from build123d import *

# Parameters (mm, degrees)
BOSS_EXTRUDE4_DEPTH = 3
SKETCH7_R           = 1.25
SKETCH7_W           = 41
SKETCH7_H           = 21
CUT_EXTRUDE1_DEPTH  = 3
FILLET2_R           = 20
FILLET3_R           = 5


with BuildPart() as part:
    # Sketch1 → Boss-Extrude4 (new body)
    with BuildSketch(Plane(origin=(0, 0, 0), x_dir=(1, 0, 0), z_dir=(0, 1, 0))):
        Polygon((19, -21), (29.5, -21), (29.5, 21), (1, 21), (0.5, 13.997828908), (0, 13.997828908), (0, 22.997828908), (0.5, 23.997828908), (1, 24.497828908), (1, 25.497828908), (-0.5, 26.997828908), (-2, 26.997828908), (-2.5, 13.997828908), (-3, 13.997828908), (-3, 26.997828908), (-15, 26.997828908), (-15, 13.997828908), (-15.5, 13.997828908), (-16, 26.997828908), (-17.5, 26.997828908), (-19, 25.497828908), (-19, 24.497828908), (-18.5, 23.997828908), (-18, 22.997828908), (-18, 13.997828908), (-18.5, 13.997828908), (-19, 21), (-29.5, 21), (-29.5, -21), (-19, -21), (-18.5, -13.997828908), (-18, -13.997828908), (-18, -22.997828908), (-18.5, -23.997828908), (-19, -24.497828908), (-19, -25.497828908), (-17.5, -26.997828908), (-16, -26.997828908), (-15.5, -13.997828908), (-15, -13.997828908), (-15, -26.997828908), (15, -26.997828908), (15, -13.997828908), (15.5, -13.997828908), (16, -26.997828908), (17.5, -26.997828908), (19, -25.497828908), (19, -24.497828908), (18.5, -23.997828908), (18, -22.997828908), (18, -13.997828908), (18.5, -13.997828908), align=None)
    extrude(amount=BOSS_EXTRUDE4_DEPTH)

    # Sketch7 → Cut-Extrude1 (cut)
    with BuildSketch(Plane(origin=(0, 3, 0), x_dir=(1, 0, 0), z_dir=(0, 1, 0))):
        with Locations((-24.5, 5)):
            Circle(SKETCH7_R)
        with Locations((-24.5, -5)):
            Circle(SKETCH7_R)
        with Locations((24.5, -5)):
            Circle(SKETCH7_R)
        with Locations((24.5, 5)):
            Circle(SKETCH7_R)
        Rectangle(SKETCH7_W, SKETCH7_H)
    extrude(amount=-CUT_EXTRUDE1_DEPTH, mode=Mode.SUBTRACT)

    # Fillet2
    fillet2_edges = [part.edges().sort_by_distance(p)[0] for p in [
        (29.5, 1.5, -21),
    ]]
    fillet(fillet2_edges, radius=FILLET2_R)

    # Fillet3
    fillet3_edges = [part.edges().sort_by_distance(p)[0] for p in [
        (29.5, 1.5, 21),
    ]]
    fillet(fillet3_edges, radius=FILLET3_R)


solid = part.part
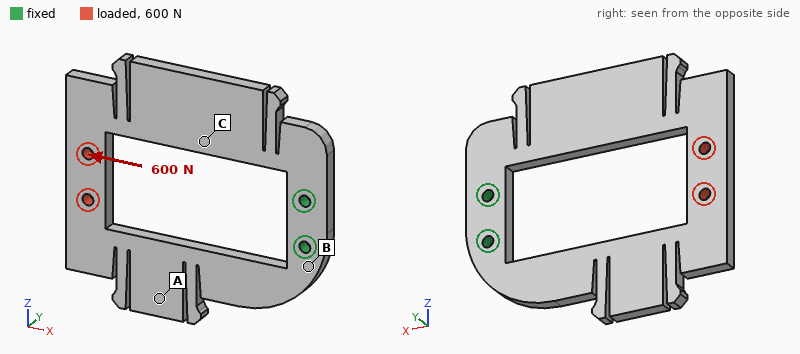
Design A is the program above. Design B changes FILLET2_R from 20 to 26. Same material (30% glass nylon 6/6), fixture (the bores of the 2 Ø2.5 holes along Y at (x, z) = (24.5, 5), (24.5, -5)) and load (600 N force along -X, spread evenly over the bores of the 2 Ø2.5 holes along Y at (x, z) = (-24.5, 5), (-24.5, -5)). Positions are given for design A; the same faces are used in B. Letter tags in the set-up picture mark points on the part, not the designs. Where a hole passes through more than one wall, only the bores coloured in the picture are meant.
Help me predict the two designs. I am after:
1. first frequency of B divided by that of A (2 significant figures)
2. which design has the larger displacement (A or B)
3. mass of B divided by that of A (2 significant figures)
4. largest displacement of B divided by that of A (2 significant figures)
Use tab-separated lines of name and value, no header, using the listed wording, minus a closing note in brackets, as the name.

first frequency of B divided by that of A	0.93
which design has the larger displacement	B
mass of B divided by that of A	0.97
largest displacement of B divided by that of A	1.6
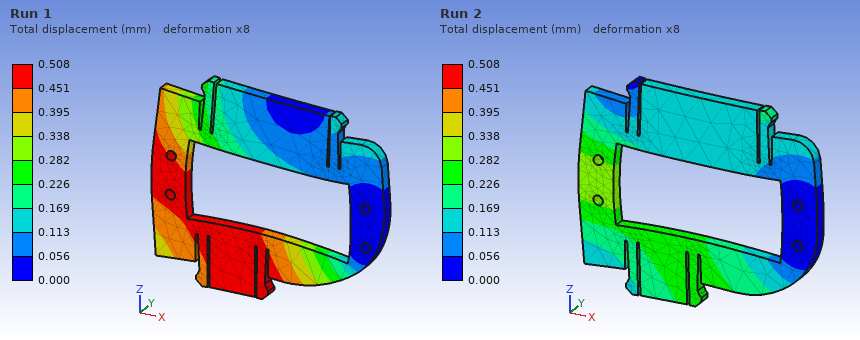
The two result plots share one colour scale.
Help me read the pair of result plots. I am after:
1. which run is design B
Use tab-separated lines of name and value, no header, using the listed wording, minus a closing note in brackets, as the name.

which run is design B	Run 1
